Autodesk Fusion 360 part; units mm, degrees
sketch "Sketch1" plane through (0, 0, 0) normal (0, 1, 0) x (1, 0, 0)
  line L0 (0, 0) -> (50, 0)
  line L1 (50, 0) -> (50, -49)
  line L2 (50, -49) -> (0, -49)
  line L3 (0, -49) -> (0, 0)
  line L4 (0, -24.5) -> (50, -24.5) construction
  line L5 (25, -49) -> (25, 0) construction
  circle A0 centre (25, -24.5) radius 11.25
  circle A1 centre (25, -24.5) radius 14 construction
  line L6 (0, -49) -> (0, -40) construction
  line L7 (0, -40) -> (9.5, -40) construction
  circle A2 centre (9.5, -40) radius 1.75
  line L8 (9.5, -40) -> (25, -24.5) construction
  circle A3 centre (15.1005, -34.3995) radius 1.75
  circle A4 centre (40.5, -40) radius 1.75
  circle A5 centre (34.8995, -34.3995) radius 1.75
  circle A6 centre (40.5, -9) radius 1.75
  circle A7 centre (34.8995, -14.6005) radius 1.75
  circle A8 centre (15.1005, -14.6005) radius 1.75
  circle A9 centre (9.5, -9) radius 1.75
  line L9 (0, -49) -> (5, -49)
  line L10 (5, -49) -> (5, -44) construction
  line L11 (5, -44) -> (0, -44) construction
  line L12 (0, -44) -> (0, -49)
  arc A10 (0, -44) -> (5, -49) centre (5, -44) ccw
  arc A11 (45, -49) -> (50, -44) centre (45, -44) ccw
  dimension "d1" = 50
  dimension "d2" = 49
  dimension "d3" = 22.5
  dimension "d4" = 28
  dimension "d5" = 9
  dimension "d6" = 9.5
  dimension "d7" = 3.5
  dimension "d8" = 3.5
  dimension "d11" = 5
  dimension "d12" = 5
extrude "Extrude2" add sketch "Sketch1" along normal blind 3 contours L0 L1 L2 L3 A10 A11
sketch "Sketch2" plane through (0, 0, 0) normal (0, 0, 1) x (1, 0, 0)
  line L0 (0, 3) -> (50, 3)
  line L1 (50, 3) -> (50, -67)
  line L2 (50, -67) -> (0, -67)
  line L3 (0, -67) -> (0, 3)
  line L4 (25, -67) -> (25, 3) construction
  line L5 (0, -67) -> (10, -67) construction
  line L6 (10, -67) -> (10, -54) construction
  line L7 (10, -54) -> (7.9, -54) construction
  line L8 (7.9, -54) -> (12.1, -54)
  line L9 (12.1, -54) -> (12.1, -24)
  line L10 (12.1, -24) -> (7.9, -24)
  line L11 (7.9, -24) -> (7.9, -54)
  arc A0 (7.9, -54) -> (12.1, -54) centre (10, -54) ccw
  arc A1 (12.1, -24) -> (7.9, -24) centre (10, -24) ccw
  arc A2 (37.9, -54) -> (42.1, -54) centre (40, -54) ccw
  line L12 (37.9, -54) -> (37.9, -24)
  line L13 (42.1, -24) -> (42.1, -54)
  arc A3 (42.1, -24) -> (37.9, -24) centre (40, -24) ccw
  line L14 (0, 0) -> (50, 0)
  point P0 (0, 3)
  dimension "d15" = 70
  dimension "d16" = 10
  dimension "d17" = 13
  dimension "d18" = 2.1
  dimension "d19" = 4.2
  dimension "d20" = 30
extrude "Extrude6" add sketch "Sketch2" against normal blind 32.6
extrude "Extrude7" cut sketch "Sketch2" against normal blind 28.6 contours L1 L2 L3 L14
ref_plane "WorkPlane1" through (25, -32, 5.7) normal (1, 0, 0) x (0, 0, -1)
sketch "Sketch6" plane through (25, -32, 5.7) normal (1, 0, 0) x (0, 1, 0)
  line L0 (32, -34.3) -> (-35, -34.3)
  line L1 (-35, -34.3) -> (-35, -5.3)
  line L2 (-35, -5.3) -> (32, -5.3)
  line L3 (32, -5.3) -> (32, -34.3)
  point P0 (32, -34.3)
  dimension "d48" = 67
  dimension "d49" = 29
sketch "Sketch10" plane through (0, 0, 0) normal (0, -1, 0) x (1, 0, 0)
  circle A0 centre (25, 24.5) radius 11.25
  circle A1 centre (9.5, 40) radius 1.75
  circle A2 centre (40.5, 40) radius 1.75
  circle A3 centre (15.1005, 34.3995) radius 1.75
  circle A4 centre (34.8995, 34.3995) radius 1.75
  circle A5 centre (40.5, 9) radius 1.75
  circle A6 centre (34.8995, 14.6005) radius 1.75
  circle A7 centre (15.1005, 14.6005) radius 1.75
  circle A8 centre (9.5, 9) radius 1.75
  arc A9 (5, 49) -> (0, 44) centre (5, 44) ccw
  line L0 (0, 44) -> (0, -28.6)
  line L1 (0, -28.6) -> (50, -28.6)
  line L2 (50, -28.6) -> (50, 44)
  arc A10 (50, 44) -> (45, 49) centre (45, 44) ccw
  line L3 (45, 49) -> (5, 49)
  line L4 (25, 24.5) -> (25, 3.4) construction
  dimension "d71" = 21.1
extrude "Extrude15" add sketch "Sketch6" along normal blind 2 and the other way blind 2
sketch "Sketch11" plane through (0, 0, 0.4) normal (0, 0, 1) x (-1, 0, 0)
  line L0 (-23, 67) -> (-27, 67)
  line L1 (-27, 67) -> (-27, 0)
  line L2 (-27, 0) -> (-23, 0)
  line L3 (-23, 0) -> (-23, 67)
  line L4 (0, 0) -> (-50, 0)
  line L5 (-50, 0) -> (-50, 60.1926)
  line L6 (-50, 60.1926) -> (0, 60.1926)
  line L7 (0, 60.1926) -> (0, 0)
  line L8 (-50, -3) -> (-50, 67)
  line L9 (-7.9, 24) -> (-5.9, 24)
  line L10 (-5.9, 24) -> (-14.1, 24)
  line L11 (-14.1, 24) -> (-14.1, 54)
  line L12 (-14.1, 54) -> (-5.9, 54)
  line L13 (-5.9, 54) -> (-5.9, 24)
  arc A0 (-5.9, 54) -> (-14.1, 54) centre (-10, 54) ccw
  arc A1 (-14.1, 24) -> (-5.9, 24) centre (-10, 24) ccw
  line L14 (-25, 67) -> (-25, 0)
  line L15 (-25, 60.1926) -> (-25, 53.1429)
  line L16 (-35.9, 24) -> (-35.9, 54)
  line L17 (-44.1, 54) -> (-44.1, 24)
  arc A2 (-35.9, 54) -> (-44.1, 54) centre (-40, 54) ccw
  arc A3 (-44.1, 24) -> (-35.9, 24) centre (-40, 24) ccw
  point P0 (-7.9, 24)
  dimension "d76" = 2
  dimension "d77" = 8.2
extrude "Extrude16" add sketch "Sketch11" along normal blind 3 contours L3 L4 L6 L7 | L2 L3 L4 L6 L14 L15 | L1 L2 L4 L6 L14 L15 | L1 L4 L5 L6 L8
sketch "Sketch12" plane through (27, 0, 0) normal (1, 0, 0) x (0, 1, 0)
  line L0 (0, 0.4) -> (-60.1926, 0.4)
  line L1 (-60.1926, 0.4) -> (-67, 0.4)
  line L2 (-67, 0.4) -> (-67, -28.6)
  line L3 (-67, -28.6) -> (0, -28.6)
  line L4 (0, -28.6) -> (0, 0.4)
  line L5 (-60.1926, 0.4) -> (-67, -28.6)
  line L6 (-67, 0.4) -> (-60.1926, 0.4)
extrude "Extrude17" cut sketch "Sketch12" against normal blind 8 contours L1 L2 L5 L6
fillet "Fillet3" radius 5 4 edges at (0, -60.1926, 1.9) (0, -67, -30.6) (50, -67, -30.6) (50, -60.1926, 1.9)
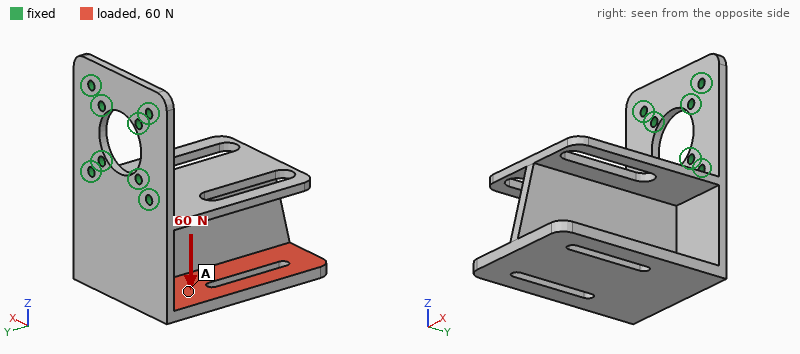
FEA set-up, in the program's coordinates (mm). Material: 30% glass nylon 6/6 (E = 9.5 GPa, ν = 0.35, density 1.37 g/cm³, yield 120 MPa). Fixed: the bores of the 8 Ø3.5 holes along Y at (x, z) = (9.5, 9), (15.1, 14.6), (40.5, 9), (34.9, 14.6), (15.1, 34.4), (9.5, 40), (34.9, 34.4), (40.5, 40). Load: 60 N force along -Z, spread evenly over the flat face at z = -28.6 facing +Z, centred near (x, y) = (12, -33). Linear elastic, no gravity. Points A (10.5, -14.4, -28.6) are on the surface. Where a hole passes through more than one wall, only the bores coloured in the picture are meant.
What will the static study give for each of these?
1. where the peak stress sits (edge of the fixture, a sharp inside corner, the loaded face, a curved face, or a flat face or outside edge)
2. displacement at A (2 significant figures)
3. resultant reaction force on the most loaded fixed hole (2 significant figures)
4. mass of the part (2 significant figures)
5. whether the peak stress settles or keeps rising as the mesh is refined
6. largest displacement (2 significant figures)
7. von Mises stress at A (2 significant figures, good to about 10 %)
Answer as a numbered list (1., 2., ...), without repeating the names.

1. edge of the fixture
2. 0.61 mm
3. 71 N
4. 52 g
5. keeps rising
6. 1.4 mm
7. 2.7 MPa
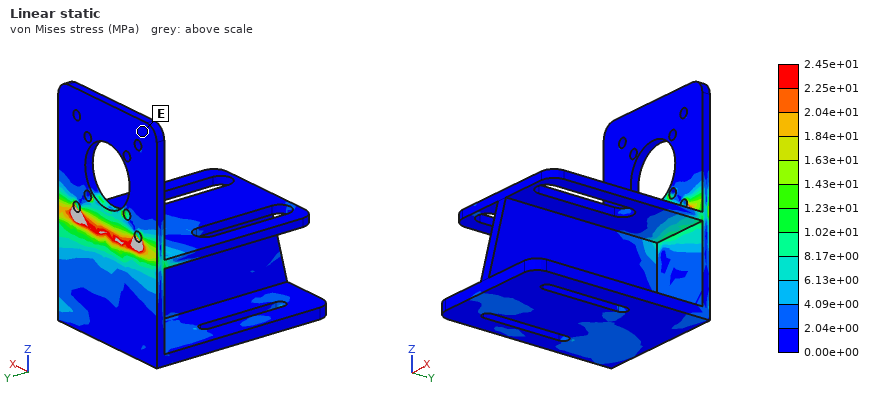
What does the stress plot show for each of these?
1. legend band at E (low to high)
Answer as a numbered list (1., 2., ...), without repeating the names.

1. 0.00e+00 to 2.04e+00 MPa
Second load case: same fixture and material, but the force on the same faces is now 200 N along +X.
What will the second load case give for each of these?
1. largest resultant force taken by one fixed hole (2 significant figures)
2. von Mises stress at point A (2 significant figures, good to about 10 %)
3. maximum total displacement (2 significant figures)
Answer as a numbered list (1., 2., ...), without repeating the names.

1. 300 N
2. 5.1 MPa
3. 1.2 mm
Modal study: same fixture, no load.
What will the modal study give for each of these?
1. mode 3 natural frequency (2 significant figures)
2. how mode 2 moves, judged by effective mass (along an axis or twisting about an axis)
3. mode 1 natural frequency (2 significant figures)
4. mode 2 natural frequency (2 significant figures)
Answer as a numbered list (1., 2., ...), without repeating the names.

1. 1500 Hz
2. along X
3. 200 Hz
4. 510 Hz
